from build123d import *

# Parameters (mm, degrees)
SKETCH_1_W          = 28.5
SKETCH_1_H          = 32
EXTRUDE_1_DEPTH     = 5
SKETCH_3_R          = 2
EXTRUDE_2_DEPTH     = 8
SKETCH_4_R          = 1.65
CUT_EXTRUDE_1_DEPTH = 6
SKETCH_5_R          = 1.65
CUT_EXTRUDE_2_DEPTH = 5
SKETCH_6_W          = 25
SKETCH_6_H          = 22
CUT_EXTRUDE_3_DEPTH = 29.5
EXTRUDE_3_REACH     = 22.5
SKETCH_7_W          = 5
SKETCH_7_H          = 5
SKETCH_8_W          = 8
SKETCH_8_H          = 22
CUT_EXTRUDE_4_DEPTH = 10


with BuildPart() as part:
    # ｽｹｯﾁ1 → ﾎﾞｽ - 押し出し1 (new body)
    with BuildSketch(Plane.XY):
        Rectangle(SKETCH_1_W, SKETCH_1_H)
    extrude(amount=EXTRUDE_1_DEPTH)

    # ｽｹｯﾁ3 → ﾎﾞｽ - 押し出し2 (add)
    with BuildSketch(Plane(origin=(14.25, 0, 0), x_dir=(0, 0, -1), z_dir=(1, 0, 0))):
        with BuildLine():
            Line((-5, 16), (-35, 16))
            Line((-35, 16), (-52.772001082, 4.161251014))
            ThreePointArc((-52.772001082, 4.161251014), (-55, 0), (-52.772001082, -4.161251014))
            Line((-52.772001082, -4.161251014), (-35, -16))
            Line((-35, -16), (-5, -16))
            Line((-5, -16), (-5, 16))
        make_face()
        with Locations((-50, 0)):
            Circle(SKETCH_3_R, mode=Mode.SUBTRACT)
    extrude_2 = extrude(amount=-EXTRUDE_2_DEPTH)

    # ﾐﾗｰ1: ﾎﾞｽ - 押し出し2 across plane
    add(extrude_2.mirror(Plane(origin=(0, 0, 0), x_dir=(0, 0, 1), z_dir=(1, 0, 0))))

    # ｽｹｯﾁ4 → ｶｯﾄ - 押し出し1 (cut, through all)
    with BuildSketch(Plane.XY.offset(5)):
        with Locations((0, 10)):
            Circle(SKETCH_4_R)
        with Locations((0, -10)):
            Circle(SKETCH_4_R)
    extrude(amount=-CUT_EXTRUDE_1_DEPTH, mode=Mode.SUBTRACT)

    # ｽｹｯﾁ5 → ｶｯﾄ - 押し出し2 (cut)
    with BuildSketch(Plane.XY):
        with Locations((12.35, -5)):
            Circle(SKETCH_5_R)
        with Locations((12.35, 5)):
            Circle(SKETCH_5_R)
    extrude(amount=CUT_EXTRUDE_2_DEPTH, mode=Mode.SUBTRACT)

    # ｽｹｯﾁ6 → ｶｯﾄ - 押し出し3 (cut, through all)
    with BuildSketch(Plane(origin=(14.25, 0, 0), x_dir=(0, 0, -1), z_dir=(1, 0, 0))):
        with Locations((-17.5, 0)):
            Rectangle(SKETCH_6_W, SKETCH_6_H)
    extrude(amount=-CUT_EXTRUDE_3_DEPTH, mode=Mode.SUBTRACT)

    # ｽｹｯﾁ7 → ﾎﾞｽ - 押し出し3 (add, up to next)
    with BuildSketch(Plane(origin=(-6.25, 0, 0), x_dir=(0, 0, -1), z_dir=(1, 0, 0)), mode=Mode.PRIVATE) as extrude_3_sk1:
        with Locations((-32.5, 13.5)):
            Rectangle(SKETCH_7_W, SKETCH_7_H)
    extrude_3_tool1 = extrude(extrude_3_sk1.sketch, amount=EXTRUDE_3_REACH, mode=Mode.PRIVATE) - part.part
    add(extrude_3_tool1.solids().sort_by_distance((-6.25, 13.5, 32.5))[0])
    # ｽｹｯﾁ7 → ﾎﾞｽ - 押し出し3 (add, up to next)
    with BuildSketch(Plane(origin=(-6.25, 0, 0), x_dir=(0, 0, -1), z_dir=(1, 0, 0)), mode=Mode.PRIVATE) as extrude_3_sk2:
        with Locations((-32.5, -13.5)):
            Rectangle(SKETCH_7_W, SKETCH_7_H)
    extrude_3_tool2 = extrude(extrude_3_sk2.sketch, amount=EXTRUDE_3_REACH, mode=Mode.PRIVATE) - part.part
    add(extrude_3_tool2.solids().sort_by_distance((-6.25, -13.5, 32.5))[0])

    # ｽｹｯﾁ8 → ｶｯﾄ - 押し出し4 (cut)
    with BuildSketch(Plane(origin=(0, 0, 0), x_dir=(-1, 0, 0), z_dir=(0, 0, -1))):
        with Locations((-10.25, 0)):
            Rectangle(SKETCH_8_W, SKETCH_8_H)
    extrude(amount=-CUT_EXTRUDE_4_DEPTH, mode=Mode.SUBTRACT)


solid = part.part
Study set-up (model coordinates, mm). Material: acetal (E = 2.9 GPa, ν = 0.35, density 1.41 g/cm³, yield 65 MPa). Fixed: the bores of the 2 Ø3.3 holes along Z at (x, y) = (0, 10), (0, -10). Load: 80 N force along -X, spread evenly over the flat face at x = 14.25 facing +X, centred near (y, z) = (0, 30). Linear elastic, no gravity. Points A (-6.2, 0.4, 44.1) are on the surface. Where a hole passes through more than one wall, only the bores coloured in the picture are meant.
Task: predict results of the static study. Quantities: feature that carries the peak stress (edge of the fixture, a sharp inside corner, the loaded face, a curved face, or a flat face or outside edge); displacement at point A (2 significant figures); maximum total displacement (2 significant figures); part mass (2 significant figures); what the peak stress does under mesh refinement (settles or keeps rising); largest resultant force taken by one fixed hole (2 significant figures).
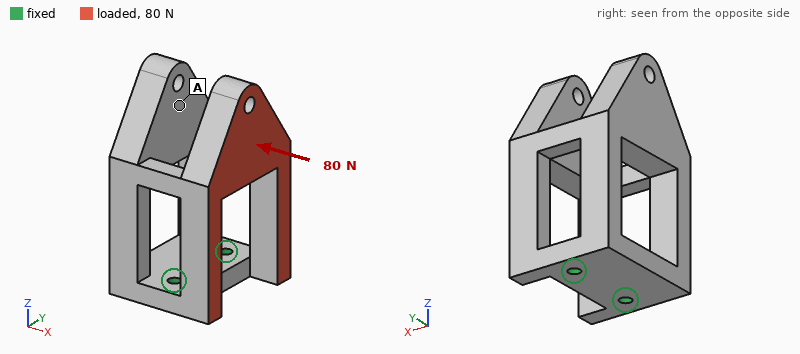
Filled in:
edge of the fixture
0.61 mm
0.82 mm
23 g
keeps rising
40 N
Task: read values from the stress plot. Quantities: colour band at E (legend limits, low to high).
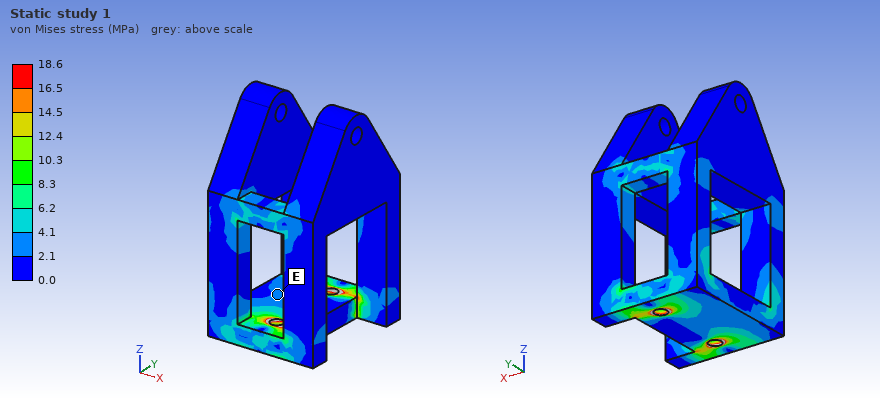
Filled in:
2.1 to 4.1 MPa
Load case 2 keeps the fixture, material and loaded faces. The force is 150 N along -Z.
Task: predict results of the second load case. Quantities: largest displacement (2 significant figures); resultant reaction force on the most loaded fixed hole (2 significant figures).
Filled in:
0.64 mm
75 N
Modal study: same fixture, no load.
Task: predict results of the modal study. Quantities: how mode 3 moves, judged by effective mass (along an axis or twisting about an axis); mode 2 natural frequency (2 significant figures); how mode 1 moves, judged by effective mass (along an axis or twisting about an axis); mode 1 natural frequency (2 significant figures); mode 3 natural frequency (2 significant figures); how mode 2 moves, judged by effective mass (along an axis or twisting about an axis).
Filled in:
twisting about Z
600 Hz
along X
440 Hz
1100 Hz
along Y
